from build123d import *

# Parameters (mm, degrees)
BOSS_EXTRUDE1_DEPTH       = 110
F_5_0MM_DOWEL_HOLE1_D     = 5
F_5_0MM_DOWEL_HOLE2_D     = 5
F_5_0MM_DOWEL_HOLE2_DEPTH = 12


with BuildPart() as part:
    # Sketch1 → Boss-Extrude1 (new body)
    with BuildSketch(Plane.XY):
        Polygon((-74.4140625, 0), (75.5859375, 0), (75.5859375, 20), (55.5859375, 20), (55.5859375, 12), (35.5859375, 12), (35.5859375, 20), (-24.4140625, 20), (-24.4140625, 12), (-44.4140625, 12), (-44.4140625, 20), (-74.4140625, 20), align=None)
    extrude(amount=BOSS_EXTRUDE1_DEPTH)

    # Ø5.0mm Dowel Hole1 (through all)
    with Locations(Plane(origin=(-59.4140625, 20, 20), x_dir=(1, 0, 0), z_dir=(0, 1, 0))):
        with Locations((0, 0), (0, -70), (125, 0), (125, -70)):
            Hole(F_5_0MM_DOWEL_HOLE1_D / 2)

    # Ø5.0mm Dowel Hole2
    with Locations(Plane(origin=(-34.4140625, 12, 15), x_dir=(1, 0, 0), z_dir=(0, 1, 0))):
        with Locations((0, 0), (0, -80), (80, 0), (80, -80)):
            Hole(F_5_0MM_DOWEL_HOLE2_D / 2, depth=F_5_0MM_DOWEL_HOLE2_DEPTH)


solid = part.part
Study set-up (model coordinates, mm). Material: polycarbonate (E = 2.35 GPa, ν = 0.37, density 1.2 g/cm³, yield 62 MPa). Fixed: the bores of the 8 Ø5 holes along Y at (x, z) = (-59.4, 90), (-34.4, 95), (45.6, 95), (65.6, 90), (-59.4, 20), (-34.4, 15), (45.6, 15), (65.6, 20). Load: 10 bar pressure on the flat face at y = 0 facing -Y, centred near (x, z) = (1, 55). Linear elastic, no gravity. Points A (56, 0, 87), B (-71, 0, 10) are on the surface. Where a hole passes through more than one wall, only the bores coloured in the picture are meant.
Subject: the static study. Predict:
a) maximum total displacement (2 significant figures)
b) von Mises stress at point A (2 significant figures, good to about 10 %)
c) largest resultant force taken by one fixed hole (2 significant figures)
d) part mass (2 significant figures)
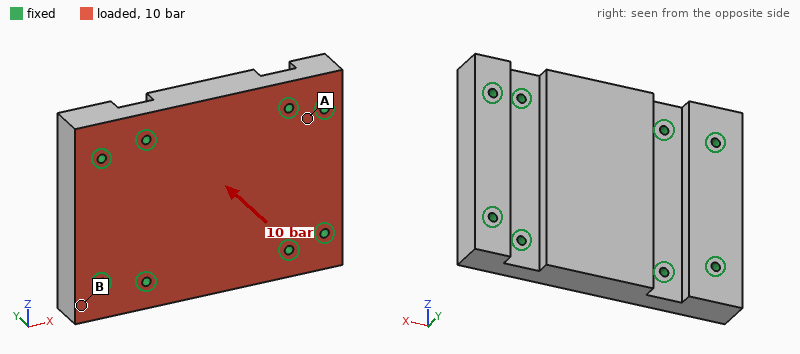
0.42 mm
8.2 MPa
2.7 kN
350 g
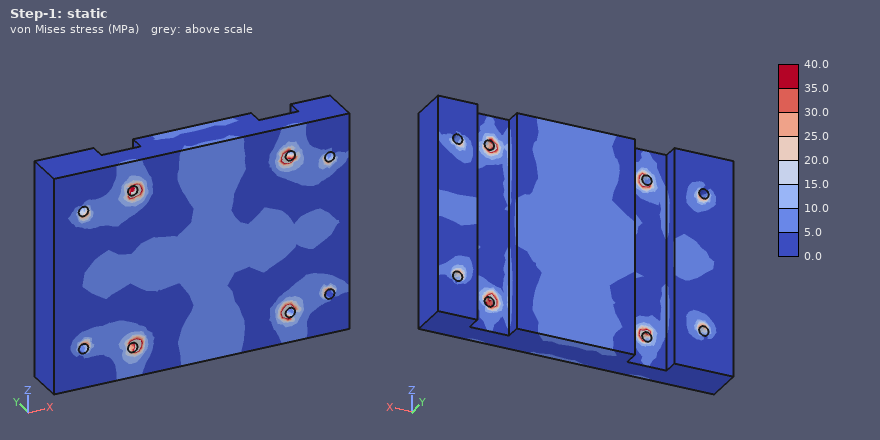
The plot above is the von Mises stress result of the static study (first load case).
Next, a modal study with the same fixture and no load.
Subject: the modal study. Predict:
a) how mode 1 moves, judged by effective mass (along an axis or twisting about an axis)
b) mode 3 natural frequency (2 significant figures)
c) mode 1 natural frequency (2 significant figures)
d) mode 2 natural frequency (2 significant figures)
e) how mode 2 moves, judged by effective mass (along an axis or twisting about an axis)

along Y
3100 Hz
1900 Hz
2500 Hz
twisting about X
